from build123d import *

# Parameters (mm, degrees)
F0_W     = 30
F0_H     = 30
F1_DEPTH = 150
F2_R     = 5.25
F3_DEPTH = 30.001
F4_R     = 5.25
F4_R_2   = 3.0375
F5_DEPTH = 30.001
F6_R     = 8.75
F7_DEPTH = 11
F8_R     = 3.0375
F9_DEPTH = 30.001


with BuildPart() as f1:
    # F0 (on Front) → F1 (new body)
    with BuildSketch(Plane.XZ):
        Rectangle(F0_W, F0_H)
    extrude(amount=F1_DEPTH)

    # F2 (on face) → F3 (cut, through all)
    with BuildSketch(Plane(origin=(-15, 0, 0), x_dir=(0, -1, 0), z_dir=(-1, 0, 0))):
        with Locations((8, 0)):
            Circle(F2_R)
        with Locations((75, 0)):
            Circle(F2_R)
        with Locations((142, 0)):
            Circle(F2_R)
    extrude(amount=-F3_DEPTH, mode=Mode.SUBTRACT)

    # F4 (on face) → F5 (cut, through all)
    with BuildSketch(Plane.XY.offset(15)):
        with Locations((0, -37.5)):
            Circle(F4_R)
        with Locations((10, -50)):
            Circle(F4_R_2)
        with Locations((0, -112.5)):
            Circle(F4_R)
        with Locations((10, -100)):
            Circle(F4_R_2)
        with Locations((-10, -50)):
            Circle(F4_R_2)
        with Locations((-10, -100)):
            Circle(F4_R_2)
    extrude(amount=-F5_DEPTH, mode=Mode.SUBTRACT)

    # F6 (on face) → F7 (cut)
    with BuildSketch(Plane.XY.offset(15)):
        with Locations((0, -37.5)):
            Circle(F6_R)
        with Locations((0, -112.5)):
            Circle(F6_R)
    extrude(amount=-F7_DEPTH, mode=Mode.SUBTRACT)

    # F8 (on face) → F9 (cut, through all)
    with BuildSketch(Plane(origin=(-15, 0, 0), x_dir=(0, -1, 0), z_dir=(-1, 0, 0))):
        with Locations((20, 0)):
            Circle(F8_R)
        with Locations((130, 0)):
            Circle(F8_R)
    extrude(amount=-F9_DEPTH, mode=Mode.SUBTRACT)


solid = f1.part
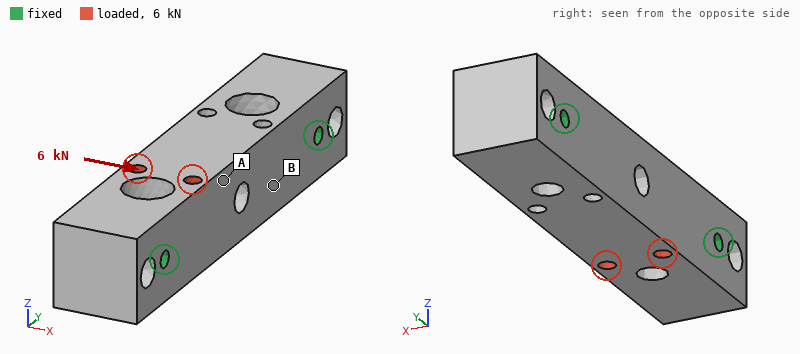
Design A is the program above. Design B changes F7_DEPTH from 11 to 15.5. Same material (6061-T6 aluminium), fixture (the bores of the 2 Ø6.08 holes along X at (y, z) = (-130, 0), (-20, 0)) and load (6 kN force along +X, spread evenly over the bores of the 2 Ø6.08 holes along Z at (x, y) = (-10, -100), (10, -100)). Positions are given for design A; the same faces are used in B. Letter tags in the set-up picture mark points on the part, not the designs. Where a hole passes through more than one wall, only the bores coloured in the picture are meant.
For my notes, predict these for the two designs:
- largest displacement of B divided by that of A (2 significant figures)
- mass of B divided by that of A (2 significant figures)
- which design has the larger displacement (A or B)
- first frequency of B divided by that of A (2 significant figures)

1.1
0.99
B
0.99
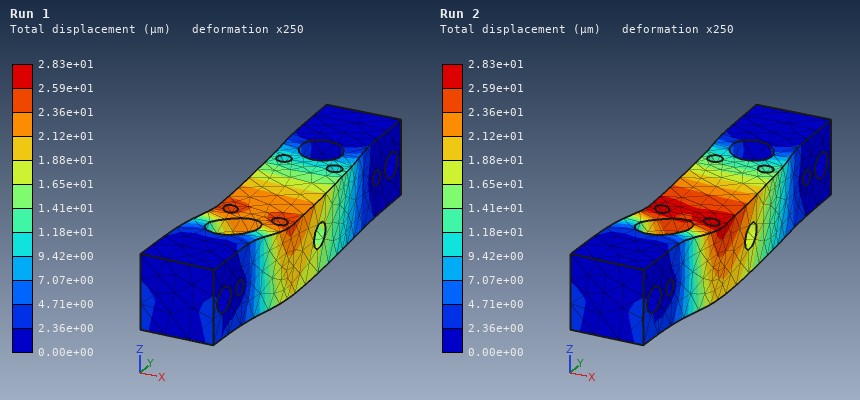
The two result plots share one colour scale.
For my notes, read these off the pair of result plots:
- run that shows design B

Run 2
